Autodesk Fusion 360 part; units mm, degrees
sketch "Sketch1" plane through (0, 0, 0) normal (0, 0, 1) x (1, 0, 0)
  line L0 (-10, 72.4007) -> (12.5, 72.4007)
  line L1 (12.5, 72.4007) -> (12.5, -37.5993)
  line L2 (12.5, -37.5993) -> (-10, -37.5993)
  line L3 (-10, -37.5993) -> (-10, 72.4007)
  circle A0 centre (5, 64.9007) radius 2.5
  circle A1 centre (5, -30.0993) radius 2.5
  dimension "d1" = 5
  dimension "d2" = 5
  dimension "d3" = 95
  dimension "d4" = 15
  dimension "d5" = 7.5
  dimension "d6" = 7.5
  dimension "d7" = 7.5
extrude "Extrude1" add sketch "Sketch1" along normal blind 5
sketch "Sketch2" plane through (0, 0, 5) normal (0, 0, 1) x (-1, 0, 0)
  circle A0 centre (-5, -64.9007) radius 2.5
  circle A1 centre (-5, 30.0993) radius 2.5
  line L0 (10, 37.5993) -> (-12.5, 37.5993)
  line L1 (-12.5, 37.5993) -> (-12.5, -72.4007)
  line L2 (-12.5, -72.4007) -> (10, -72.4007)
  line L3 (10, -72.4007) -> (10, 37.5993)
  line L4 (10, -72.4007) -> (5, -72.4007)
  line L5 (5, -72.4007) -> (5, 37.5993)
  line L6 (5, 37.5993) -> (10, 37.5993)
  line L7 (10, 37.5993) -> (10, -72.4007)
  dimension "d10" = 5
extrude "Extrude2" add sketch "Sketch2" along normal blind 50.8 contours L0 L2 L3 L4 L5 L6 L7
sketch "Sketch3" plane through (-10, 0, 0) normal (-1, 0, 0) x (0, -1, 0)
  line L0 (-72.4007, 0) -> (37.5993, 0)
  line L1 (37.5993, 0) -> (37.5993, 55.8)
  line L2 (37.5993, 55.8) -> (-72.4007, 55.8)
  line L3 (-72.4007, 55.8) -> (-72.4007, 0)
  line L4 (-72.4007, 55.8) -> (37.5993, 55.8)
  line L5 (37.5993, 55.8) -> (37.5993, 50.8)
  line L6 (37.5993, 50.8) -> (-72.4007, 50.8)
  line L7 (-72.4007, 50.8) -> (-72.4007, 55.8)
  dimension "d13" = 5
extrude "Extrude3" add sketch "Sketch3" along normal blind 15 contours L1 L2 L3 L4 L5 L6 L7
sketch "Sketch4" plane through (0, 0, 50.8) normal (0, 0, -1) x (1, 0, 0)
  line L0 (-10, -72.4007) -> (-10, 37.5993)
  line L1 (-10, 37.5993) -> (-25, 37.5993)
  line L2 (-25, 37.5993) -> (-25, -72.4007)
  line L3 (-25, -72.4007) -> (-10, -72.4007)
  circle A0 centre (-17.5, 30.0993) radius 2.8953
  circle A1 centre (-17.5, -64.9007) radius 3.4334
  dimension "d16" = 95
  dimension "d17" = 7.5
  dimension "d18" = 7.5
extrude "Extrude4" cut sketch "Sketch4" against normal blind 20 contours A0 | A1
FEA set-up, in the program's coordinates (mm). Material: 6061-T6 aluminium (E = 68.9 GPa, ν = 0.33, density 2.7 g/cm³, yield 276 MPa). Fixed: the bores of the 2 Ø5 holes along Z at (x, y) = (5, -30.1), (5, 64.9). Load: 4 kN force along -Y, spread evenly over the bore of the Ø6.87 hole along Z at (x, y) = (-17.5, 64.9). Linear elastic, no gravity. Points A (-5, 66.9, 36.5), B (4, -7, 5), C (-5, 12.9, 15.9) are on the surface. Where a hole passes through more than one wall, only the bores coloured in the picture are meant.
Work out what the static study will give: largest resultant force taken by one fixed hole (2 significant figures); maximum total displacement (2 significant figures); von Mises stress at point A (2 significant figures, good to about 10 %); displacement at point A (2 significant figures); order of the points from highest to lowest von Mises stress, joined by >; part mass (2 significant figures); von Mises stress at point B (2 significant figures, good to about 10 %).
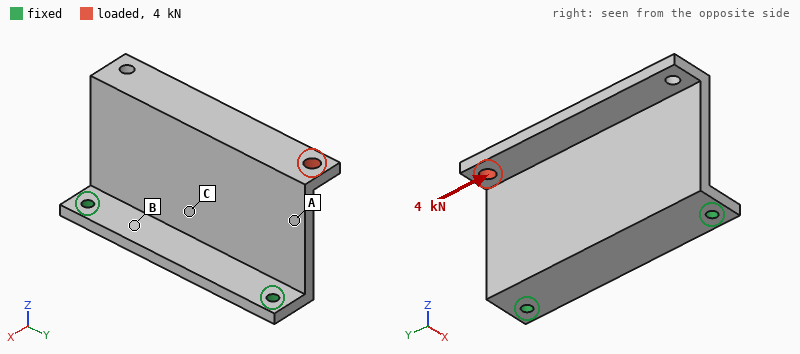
3.1 kN
0.41 mm
47 MPa
0.18 mm
A > B > C
130 g
29 MPa
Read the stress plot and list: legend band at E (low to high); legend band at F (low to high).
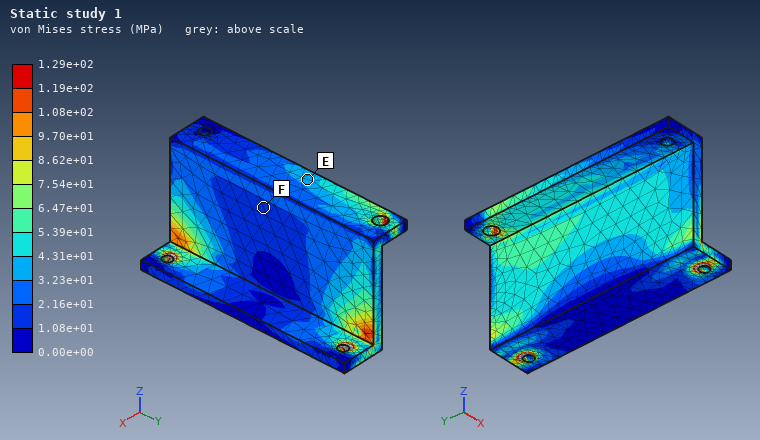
3.23e+01 to 4.31e+01 MPa
1.08e+01 to 2.16e+01 MPa
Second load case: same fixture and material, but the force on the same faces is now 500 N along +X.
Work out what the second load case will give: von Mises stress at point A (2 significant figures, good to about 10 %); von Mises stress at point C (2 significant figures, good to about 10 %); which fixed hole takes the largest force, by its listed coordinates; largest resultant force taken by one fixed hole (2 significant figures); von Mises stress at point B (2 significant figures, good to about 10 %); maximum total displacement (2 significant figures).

41 MPa
34 MPa
(5, 64.9)
520 N
43 MPa
1.1 mm
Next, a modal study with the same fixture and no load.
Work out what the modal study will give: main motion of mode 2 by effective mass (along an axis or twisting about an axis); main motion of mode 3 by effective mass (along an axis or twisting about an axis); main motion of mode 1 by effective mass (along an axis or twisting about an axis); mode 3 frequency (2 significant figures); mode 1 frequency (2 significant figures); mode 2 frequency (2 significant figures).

twisting about Z
along Y
along X
3800 Hz
620 Hz
1500 Hz
